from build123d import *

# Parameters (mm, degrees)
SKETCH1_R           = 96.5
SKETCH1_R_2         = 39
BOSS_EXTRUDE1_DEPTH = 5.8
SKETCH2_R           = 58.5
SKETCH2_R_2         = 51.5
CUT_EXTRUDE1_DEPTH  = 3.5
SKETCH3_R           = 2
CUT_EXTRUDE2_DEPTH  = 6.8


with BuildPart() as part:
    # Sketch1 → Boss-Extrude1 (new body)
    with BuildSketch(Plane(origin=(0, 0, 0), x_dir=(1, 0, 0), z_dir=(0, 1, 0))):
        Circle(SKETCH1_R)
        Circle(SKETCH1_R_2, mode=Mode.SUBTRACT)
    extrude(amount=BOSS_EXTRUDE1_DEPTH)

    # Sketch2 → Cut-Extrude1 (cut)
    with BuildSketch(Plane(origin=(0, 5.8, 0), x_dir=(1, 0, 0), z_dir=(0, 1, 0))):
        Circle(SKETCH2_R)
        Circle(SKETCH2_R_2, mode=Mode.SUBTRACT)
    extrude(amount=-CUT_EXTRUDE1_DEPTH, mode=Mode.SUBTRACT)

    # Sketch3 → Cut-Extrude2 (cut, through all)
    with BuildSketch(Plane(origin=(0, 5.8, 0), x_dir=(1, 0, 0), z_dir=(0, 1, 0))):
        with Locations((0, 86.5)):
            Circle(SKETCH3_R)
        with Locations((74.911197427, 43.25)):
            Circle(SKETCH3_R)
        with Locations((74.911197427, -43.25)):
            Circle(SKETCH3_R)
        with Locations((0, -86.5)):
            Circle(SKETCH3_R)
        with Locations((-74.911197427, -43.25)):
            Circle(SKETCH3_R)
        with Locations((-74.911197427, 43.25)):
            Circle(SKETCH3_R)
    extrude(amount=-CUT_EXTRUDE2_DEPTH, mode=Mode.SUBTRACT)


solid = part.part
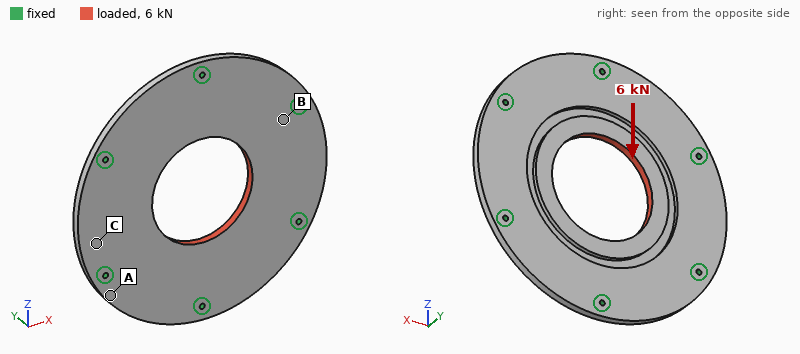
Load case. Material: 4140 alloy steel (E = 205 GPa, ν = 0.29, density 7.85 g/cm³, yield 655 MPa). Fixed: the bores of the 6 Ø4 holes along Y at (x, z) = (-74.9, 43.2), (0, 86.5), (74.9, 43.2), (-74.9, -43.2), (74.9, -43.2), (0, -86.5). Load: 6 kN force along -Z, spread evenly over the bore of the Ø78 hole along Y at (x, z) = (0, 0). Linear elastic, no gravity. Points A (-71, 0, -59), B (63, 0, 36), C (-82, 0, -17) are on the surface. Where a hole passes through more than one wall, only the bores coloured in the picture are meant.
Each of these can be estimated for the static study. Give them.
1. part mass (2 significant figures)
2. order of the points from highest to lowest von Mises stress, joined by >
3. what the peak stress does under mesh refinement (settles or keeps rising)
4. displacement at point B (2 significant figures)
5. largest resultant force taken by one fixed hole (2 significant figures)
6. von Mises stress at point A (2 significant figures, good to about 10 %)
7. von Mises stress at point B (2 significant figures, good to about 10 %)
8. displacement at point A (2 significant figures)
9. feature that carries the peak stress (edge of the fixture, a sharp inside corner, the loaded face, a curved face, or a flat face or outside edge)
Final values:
1.0 kg
B > A > C
keeps rising
1.0 µm
1.3 kN
4.0 MPa
6.5 MPa
0.91 µm
edge of the fixture
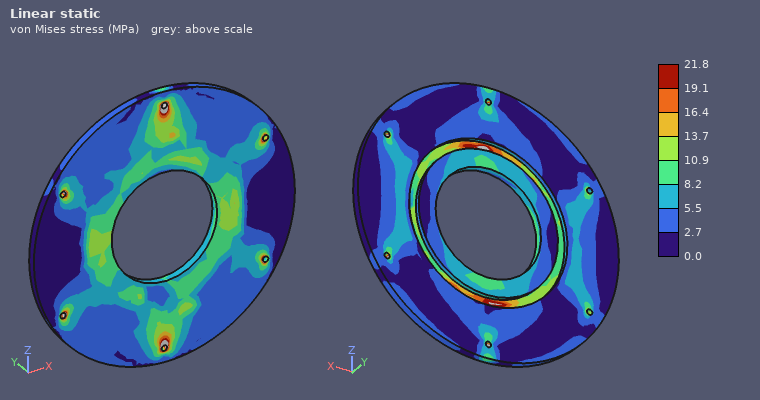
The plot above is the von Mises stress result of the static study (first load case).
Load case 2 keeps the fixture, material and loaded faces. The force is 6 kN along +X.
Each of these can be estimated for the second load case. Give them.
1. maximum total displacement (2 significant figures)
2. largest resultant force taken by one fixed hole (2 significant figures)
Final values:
5.6 µm
1.2 kN
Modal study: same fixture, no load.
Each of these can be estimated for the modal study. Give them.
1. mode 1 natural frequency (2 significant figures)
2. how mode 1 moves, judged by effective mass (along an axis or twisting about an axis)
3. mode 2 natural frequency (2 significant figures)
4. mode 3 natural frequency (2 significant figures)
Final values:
2000 Hz
along Y
2700 Hz
2700 Hz
